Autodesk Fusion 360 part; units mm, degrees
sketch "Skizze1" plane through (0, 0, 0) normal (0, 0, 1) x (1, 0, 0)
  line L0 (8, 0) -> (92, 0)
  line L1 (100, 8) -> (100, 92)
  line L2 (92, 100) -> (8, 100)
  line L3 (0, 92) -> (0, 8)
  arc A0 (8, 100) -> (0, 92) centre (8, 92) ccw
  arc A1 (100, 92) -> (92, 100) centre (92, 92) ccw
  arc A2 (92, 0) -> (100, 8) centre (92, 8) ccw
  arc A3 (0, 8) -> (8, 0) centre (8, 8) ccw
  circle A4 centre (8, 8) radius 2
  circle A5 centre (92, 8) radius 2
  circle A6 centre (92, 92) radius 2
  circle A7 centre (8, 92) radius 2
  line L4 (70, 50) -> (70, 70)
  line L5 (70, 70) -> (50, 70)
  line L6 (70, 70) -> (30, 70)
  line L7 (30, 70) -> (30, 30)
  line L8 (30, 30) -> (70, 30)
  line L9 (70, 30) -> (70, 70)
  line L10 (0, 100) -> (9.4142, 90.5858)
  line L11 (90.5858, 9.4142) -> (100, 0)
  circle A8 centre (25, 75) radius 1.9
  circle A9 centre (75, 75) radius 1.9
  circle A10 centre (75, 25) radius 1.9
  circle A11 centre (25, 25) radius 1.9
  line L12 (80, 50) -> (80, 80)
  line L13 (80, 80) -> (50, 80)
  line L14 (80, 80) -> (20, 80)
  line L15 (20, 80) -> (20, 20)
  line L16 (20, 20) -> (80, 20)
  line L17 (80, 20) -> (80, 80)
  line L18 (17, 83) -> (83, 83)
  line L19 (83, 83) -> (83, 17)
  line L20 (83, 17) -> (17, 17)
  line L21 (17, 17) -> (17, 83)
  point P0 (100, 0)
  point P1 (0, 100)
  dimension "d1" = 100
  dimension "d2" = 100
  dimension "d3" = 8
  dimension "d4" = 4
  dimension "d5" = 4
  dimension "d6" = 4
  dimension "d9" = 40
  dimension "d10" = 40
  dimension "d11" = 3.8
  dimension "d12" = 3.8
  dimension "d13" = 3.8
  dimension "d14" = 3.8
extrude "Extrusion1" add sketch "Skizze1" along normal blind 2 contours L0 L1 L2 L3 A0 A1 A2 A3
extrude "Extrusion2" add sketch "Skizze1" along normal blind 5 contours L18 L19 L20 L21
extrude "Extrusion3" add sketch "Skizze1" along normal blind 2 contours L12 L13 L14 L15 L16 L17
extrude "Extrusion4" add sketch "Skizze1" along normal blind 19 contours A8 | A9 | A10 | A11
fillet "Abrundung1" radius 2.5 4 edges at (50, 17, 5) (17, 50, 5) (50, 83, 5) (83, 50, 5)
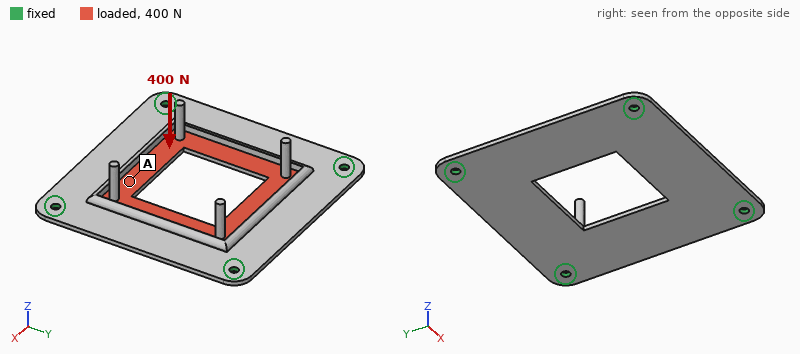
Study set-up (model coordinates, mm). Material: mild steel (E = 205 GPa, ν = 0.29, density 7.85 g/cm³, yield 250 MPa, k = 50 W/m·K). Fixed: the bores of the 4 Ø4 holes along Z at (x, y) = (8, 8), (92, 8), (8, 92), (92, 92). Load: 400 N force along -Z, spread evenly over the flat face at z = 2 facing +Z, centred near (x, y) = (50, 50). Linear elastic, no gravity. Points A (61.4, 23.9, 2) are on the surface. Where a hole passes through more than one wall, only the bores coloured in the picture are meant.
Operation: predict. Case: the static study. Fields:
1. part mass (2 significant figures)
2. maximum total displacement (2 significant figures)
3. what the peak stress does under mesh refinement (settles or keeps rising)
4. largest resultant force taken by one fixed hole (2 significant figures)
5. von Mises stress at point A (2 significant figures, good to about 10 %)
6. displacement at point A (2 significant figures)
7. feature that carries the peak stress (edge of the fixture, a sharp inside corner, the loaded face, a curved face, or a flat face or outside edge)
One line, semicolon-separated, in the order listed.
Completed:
150 g; 0.12 mm; keeps rising; 220 N; 20 MPa; 0.087 mm; edge of the fixture
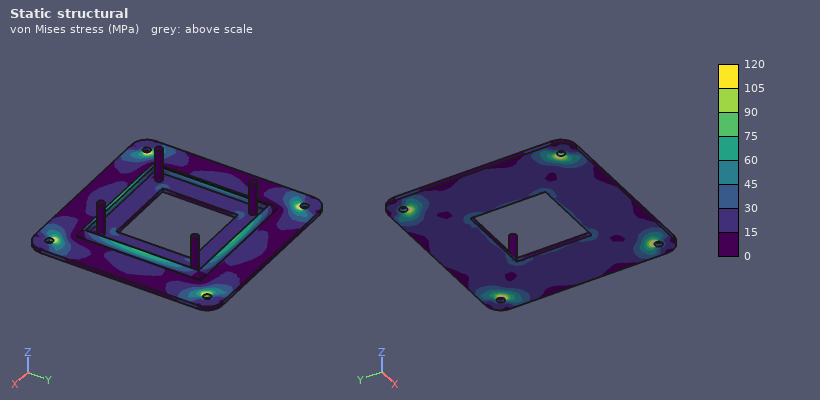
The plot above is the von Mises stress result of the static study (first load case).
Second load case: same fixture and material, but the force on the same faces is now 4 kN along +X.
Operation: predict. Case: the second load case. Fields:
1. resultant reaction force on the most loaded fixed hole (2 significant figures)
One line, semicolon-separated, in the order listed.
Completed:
1.1 kN
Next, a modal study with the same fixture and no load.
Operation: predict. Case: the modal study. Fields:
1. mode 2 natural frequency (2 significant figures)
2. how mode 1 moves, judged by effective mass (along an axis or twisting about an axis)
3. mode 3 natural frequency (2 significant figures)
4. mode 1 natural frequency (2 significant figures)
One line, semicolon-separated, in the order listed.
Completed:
1900 Hz; along Z; 1900 Hz; 1300 Hz
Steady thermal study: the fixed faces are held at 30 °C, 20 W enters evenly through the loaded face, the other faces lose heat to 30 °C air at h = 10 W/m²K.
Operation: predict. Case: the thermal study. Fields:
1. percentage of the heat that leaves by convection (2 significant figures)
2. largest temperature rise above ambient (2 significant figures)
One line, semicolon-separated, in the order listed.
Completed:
23 %; 40 K
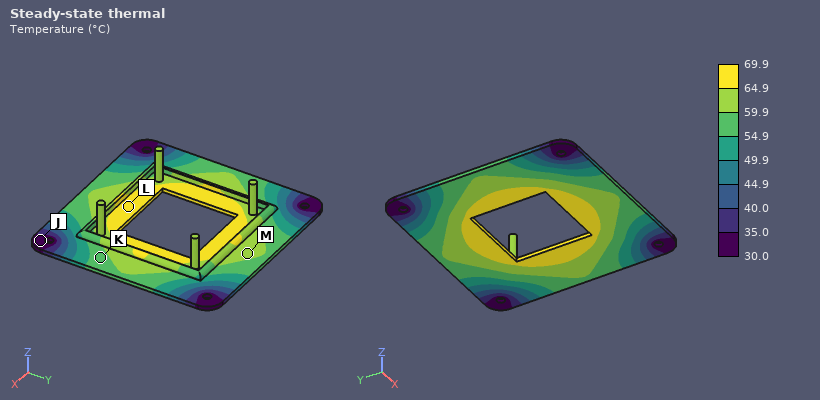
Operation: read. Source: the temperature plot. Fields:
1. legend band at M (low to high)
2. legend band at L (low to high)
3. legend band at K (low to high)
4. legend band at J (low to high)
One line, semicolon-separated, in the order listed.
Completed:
59.9 to 64.9 °C; 64.9 to 69.9 °C; 54.9 to 59.9 °C; 30.0 to 35.0 °C
